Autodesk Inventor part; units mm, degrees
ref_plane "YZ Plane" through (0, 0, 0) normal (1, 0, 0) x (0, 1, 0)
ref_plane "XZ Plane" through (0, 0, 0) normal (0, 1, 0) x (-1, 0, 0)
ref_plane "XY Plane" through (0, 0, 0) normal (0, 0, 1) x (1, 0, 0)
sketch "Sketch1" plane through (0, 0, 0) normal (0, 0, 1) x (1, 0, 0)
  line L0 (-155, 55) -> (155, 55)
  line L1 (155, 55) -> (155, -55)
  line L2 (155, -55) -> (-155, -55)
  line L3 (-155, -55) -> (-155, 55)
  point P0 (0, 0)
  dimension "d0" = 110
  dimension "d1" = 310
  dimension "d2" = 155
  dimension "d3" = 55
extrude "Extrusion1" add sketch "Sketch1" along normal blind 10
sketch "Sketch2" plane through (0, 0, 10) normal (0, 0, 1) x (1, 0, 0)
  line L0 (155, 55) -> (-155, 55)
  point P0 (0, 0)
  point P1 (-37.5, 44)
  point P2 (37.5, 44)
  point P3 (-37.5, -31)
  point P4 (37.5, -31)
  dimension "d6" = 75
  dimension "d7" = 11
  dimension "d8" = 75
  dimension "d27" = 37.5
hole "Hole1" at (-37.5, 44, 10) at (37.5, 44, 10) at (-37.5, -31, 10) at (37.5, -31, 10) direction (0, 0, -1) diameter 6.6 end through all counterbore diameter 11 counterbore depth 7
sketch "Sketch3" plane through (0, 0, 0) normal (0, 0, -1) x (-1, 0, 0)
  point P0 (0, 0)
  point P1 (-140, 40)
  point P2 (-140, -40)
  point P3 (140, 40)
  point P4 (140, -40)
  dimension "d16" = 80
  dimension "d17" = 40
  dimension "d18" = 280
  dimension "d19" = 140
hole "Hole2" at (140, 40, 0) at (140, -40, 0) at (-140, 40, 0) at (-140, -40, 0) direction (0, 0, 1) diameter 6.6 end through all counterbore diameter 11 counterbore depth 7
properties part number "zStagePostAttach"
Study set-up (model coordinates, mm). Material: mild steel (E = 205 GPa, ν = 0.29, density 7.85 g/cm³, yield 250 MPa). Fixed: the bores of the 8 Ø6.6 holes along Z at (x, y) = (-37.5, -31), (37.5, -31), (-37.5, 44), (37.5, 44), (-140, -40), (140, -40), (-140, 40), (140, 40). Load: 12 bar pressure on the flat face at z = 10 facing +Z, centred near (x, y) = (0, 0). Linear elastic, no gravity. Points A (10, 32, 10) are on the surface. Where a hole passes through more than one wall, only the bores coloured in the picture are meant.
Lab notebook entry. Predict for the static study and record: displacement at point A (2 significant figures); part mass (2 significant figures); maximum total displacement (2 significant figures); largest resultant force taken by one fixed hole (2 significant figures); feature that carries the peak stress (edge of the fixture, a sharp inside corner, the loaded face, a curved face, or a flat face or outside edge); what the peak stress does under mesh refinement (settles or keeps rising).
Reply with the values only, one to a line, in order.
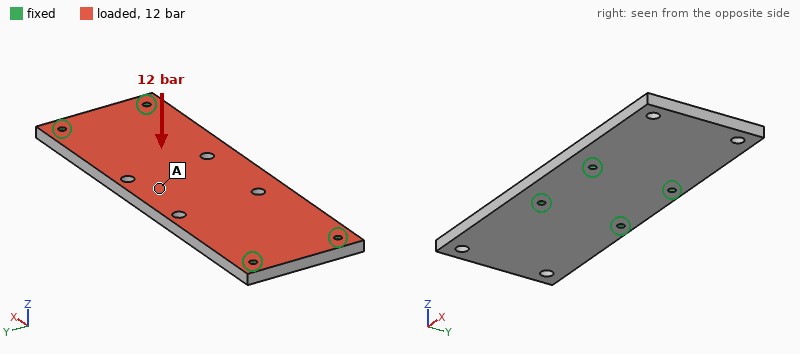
11 µm
2.6 kg
55 µm
7.4 kN
edge of the fixture
keeps rising
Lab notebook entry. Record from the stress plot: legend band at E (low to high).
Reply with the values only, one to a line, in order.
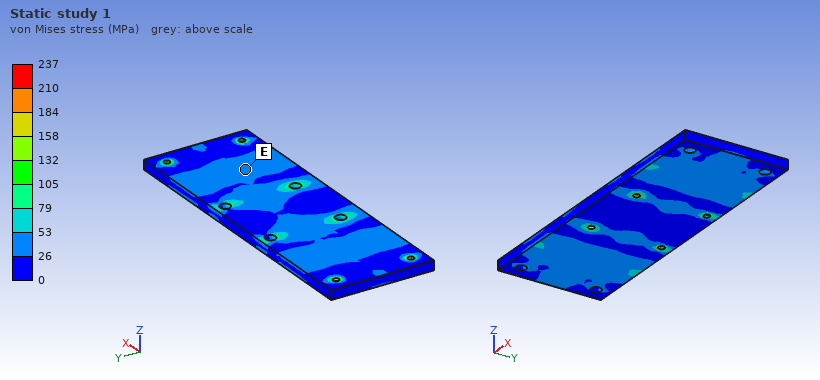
26 to 53 MPa
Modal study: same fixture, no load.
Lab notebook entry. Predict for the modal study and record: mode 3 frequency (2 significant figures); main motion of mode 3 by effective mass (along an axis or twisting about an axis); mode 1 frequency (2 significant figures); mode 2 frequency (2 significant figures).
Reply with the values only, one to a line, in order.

4100 Hz
twisting about X
2900 Hz
2900 Hz
